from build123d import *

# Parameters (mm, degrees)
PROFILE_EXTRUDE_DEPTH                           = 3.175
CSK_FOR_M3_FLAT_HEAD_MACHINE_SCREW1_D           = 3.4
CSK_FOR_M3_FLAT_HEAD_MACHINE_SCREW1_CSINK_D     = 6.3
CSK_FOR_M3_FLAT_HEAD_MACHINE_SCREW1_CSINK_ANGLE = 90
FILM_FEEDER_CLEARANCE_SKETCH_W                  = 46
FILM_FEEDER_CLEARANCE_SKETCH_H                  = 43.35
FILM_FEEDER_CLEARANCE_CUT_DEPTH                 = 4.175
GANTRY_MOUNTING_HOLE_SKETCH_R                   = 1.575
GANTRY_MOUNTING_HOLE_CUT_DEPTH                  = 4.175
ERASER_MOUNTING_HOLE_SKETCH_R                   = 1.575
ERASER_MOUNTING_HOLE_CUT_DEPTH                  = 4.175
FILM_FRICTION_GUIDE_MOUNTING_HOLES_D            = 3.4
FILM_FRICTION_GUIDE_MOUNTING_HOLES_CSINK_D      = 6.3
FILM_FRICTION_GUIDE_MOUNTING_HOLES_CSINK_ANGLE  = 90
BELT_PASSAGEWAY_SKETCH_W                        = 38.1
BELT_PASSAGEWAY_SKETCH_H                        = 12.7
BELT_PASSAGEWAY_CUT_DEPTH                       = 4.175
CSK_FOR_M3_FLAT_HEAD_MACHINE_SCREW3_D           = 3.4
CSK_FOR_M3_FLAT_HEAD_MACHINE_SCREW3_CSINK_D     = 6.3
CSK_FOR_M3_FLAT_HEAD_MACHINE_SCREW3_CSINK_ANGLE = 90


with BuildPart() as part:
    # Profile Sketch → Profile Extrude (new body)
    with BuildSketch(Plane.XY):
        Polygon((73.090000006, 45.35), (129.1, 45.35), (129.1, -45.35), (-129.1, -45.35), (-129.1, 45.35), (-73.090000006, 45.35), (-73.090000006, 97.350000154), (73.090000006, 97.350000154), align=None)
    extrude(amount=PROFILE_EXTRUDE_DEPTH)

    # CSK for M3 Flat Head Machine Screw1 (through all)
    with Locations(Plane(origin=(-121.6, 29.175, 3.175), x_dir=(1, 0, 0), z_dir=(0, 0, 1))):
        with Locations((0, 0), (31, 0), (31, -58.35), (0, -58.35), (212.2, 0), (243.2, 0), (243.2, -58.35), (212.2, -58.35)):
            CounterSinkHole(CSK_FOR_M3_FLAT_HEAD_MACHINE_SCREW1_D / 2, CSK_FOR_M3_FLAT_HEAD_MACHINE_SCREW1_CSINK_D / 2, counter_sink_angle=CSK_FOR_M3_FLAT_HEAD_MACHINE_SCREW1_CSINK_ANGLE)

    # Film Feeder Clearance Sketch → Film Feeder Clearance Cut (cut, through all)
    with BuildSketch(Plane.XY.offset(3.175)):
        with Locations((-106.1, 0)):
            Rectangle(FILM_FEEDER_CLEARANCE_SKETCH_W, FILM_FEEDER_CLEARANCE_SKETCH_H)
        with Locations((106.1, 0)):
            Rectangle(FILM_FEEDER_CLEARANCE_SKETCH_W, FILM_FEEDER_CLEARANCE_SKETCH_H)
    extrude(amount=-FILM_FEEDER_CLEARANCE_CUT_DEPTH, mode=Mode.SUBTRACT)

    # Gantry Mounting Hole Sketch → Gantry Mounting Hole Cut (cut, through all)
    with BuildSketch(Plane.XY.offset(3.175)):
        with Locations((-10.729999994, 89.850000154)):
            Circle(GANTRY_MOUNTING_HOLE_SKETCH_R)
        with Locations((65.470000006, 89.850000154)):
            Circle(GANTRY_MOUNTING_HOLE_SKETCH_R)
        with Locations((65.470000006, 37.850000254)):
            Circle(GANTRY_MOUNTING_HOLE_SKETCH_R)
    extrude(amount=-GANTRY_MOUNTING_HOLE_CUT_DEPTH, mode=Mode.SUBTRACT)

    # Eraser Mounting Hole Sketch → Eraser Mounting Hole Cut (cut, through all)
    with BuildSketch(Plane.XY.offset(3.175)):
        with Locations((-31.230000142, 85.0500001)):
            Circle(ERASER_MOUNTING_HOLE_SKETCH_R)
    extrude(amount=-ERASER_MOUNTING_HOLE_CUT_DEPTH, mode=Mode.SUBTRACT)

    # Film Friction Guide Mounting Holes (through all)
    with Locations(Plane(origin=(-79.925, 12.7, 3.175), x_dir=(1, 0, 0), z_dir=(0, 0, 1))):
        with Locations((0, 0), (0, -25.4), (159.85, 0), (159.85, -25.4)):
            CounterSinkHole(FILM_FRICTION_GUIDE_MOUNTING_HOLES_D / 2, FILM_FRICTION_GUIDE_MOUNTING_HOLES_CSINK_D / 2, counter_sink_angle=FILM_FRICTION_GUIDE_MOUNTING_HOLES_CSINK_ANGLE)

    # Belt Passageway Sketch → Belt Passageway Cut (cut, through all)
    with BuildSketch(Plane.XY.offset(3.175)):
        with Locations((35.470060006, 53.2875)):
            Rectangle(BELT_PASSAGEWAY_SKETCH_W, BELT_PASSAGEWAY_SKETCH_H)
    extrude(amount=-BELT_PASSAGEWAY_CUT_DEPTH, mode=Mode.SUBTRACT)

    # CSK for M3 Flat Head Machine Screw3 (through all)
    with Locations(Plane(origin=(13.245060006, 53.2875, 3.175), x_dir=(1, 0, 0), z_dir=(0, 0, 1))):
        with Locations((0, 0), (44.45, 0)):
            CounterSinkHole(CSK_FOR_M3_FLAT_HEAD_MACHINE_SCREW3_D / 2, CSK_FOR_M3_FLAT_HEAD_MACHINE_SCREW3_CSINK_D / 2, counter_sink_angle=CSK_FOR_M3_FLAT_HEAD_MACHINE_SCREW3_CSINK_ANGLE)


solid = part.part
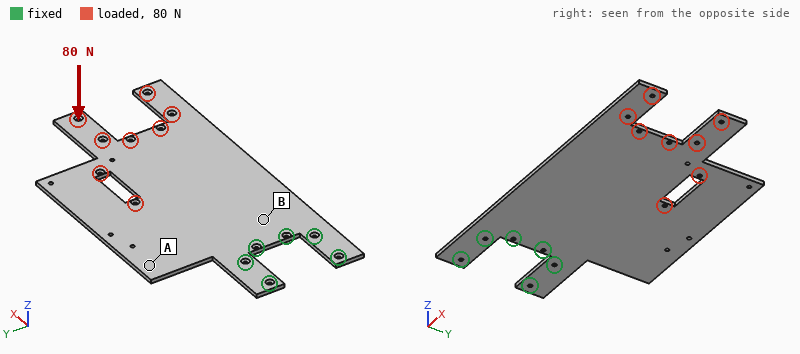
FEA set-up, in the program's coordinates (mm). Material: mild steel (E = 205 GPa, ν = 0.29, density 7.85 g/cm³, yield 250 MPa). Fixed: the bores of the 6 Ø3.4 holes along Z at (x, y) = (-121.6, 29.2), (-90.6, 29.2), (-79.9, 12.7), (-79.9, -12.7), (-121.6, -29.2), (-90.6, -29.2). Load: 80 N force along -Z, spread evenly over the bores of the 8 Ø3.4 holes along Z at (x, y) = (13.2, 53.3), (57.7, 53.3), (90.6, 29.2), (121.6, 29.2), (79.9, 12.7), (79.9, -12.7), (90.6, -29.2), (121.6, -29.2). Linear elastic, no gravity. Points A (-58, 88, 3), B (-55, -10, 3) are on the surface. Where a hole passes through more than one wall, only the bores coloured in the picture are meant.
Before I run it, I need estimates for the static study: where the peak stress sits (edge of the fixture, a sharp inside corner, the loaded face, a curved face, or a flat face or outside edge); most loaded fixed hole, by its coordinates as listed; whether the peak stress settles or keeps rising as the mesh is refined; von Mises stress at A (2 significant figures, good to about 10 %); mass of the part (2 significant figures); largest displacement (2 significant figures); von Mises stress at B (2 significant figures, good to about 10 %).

edge of the fixture
(-79.9, 12.7)
keeps rising
14 MPa
660 g
2.9 mm
56 MPa
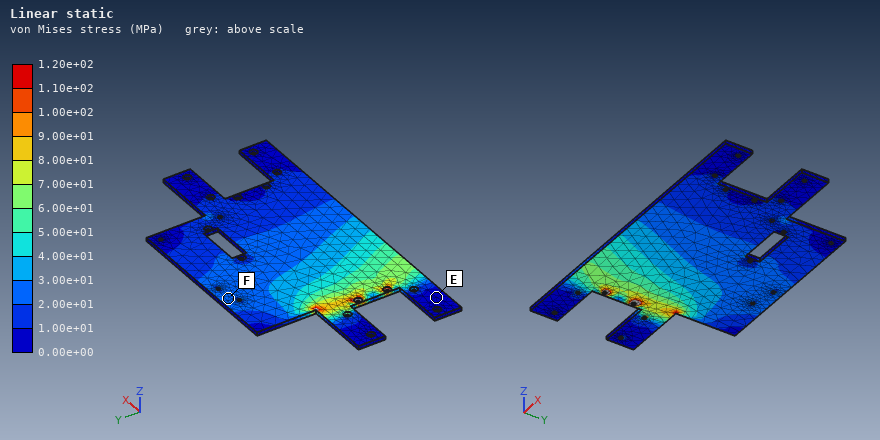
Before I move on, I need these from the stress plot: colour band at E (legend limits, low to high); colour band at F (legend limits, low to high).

0.00e+00 to 1.00e+01 MPa
2.00e+01 to 3.00e+01 MPa
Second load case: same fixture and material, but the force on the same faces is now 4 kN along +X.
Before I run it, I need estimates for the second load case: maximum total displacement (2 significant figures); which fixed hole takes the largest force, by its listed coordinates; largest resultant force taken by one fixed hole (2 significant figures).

0.96 mm
(-90.6, 29.2)
1.4 kN
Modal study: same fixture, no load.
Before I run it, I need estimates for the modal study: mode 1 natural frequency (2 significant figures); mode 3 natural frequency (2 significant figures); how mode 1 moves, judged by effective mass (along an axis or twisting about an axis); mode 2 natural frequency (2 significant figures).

68 Hz
380 Hz
along Z
180 Hz
